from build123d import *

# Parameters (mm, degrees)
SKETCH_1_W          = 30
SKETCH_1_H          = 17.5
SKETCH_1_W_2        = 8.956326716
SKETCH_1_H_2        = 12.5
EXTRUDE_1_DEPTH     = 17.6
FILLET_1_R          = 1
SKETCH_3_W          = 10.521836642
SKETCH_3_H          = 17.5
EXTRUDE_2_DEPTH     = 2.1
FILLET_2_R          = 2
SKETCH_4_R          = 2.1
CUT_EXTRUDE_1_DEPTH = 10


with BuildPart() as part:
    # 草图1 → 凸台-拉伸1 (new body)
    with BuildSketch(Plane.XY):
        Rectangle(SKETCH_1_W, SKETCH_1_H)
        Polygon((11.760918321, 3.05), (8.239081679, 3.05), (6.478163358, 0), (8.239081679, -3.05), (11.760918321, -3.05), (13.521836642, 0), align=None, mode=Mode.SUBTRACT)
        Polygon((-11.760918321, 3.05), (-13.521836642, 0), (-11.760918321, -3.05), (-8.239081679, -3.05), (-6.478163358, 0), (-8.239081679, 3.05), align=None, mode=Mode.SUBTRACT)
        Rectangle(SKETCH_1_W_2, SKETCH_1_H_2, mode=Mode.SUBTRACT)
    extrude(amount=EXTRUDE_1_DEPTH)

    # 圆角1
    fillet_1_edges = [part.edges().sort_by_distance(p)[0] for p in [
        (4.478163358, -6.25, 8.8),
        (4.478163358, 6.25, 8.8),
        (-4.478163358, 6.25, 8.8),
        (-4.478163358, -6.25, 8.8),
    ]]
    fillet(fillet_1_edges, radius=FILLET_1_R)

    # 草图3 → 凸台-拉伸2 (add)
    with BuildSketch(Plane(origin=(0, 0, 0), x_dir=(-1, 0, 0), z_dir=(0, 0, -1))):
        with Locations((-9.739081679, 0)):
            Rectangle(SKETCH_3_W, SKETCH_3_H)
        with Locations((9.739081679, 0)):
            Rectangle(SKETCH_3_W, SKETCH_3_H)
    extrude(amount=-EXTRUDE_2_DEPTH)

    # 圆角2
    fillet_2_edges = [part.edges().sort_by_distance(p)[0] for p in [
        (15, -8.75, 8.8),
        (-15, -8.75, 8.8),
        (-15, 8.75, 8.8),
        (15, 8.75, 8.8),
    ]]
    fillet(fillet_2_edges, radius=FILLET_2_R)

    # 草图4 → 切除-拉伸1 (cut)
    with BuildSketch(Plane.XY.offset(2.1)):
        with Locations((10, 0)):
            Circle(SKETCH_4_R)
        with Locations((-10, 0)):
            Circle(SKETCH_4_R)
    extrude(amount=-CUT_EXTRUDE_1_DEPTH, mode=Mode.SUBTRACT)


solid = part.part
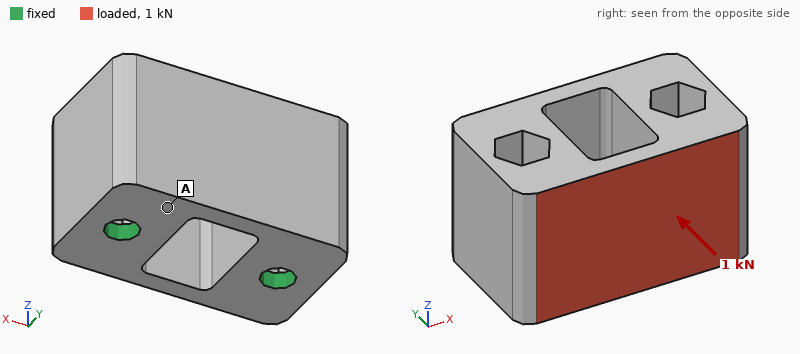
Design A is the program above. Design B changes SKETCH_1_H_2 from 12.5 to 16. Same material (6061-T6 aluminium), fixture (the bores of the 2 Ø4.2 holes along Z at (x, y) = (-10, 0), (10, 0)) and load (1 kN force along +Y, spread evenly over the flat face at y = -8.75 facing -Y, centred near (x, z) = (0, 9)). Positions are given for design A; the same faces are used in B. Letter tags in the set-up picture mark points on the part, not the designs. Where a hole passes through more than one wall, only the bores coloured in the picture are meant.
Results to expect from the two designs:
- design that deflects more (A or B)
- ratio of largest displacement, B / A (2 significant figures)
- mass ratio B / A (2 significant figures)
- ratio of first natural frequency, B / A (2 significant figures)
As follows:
B
1.3
0.91
1.0
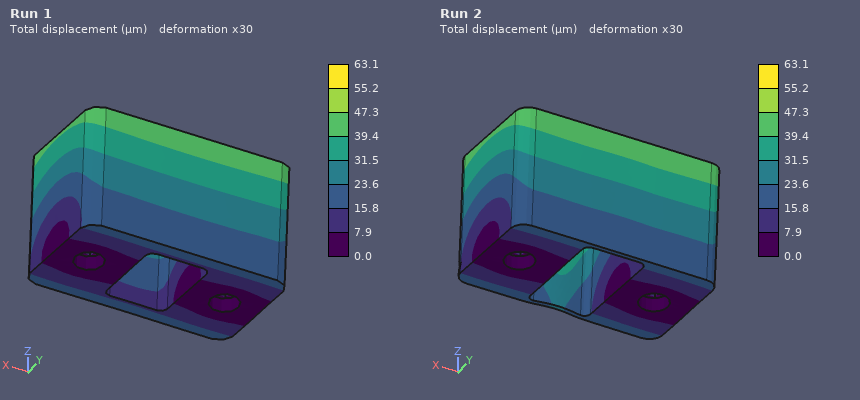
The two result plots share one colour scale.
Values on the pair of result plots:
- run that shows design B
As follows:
Run 2
